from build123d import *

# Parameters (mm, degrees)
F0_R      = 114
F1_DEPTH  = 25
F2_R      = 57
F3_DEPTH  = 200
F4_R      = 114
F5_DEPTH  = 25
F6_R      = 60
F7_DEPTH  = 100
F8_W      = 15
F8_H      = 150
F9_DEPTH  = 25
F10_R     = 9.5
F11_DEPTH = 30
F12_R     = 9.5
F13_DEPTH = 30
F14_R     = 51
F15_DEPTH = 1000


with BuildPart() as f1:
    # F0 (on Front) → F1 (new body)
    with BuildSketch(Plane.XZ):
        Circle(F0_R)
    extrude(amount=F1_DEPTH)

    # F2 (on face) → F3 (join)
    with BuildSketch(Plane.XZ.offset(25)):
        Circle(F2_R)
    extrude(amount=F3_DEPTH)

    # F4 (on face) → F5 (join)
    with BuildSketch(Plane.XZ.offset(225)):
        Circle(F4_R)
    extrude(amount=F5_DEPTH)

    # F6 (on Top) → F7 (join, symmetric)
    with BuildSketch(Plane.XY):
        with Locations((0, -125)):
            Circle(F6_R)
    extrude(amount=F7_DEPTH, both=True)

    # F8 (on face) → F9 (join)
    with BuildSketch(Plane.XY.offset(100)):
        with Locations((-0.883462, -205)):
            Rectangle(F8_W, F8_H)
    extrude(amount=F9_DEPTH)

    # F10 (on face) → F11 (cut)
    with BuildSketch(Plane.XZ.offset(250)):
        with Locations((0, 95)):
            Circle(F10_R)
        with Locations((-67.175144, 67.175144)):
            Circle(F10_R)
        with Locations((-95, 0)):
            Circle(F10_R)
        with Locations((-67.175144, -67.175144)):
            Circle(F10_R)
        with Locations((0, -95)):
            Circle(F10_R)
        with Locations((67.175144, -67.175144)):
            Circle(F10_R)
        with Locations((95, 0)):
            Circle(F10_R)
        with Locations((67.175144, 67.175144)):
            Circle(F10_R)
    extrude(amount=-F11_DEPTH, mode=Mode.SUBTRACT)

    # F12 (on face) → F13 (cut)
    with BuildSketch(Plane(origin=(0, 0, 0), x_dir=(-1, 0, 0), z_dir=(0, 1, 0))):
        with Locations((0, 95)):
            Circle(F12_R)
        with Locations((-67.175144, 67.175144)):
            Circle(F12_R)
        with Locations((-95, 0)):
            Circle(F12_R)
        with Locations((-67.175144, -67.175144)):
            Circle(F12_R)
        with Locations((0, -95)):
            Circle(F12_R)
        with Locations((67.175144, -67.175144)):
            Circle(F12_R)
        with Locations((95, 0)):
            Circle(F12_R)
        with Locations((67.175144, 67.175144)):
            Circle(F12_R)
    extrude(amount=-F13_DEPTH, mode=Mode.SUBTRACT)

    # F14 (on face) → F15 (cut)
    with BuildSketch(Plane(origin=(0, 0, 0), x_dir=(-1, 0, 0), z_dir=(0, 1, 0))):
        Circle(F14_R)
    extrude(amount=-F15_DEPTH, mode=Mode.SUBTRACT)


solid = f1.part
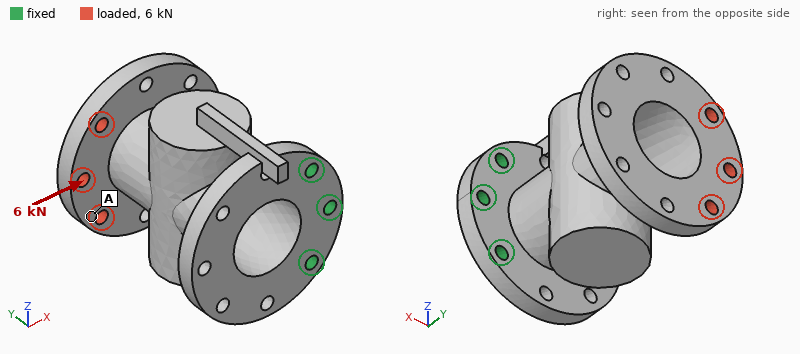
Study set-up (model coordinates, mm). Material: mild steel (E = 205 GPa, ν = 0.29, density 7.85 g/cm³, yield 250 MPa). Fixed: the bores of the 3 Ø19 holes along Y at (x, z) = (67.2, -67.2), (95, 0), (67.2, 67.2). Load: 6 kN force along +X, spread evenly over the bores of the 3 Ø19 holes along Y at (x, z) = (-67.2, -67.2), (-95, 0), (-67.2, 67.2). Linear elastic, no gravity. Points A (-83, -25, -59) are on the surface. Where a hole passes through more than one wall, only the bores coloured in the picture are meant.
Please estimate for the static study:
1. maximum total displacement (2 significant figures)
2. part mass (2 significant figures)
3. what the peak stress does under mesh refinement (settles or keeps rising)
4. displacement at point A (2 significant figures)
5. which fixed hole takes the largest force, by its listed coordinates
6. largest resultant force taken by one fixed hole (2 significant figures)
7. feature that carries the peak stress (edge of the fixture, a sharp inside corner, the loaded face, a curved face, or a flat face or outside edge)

0.50 mm
25 kg
keeps rising
0.43 mm
(95, 0)
14 kN
edge of the fixture
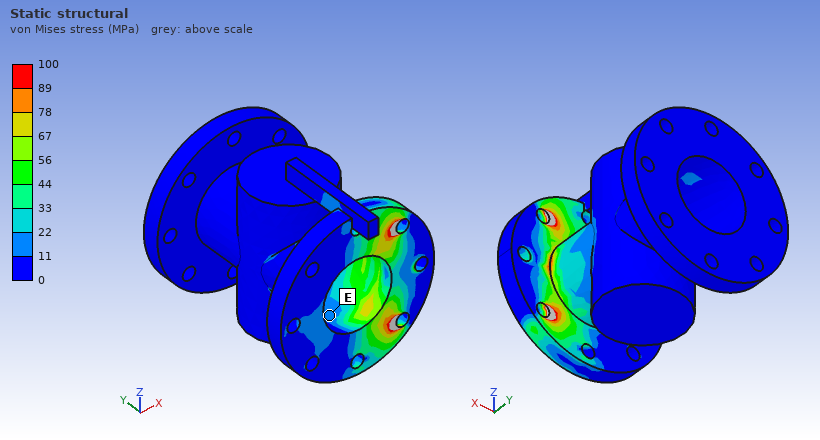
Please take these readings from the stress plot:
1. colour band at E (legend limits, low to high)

11 to 22 MPa
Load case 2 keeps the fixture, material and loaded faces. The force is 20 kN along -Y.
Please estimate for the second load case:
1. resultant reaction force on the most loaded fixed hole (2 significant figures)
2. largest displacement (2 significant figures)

21 kN
0.97 mm
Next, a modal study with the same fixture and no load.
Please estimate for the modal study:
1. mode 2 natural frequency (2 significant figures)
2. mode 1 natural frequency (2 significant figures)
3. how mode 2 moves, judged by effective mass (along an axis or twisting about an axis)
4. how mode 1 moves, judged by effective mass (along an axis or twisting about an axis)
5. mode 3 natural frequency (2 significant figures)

380 Hz
180 Hz
along Z
along X
930 Hz
